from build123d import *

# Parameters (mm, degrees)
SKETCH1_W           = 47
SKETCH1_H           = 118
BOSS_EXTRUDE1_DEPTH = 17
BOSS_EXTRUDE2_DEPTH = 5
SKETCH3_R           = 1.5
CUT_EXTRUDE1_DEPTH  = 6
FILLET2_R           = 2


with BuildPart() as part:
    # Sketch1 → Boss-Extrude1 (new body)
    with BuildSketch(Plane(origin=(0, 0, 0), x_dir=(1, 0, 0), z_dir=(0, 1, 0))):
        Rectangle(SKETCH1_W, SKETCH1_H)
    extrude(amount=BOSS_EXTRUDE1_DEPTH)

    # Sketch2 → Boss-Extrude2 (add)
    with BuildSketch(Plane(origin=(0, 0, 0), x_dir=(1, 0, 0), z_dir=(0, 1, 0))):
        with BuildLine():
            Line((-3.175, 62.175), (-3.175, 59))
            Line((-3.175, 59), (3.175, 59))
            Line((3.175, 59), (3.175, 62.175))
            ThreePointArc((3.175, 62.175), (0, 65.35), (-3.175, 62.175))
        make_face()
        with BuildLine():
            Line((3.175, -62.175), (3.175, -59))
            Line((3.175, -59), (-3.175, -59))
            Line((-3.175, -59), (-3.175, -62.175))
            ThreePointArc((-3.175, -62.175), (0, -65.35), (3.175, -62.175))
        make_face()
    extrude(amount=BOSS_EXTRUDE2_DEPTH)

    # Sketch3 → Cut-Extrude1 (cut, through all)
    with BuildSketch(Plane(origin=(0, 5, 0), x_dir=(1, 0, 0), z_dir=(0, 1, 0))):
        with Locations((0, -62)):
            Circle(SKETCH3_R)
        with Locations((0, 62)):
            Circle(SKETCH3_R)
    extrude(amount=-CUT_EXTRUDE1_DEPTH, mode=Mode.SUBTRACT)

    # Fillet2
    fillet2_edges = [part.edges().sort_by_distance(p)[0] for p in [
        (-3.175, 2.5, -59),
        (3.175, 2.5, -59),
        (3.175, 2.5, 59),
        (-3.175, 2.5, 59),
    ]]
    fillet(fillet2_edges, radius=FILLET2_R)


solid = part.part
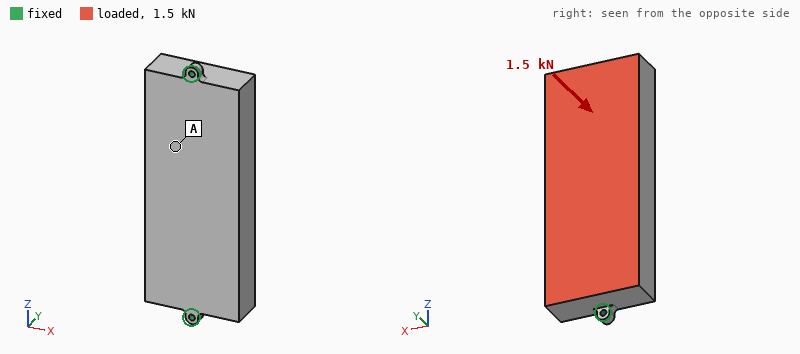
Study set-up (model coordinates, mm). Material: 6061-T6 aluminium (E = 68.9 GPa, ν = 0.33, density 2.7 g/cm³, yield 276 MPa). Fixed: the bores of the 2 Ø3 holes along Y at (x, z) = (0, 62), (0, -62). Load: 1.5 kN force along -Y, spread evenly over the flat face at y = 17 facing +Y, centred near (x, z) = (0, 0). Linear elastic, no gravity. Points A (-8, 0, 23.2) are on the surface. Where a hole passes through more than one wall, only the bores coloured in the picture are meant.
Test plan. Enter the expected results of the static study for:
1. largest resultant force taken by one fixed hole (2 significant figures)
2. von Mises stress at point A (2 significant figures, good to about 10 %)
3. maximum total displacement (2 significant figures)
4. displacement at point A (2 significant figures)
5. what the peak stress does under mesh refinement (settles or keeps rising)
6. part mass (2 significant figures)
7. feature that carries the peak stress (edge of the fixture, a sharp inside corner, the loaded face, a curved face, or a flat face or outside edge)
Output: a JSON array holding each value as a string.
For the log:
["1.1 kN", "4.9 MPa", "24 µm", "20 µm", "keeps rising", "260 g", "edge of the fixture"]
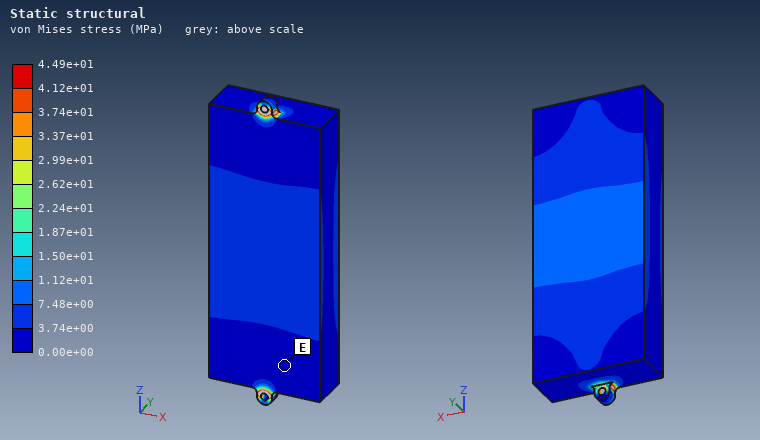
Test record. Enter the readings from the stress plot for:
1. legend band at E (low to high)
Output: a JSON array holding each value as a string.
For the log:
["0.00e+00 to 3.74e+00 MPa"]
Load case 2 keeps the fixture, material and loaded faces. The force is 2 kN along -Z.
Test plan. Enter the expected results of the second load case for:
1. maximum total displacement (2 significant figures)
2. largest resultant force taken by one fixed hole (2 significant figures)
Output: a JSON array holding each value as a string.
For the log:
["4.3 µm", "1.0 kN"]
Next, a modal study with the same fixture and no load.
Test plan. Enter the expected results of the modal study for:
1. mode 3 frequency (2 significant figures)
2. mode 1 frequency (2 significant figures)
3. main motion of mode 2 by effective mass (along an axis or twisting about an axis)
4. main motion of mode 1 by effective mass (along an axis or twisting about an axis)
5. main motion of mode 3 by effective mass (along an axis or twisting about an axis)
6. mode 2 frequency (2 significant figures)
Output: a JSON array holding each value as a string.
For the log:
["4900 Hz", "1000 Hz", "along Y", "along X", "along X", "2800 Hz"]
